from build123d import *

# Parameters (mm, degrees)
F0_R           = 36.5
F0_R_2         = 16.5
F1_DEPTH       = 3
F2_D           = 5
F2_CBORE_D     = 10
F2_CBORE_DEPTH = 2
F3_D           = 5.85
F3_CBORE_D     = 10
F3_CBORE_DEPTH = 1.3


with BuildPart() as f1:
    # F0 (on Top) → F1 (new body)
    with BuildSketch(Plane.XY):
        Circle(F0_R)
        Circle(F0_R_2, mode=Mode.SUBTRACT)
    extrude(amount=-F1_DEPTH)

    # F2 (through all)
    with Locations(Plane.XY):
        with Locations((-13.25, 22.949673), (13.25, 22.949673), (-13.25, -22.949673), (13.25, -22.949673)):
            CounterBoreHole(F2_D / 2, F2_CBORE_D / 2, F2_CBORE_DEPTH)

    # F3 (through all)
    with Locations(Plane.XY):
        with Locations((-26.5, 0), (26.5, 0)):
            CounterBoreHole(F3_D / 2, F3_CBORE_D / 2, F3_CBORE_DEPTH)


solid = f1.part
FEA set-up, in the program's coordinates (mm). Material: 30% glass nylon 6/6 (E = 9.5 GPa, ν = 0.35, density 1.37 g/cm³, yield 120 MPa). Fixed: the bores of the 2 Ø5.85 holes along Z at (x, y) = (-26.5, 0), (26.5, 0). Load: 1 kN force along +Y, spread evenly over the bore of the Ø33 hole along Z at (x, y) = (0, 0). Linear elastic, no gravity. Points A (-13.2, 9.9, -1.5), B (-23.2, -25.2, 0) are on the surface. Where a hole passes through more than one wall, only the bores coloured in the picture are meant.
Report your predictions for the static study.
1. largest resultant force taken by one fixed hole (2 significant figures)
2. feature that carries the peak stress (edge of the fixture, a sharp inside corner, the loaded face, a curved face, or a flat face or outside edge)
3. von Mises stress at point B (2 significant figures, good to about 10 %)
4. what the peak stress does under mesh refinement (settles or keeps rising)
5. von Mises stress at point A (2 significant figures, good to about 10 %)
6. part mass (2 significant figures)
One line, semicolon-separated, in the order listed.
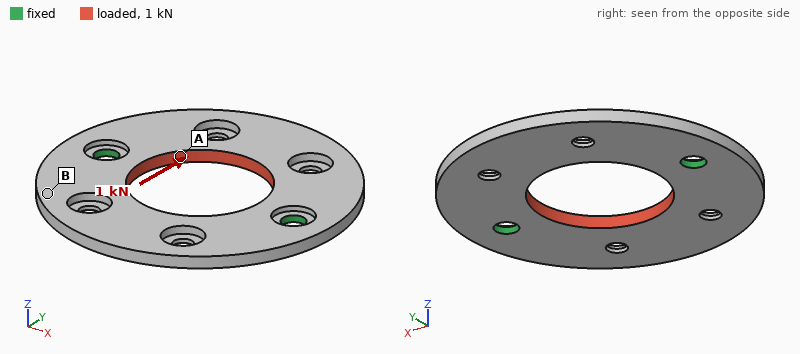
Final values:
500 N; edge of the fixture; 3.8 MPa; keeps rising; 9.8 MPa; 12 g
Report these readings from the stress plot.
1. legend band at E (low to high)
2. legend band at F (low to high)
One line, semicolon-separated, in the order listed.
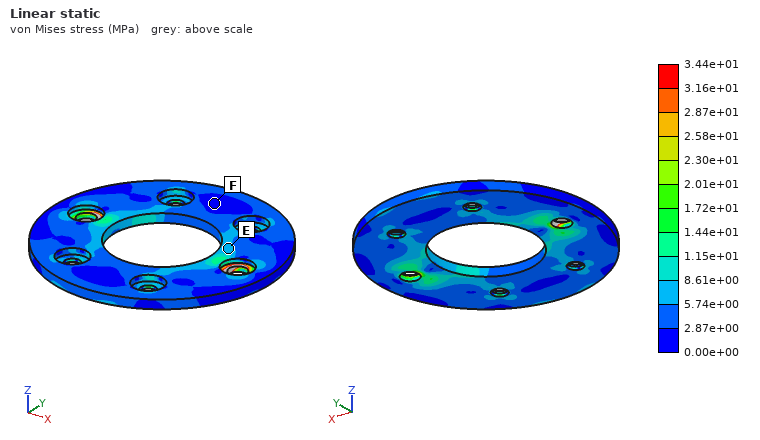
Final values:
5.74e+00 to 8.61e+00 MPa; 0.00e+00 to 2.87e+00 MPa
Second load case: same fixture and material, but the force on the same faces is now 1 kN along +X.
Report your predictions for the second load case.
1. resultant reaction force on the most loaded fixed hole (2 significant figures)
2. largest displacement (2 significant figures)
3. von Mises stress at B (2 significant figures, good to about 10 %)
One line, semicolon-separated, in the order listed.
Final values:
500 N; 35 µm; 2.3 MPa
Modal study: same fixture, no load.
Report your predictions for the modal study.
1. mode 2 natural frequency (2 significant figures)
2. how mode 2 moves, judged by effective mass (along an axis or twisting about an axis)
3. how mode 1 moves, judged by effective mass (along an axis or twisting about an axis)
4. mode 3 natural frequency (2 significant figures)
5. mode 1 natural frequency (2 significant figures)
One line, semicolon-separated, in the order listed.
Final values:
890 Hz; along Z; twisting about X; 2000 Hz; 780 Hz
